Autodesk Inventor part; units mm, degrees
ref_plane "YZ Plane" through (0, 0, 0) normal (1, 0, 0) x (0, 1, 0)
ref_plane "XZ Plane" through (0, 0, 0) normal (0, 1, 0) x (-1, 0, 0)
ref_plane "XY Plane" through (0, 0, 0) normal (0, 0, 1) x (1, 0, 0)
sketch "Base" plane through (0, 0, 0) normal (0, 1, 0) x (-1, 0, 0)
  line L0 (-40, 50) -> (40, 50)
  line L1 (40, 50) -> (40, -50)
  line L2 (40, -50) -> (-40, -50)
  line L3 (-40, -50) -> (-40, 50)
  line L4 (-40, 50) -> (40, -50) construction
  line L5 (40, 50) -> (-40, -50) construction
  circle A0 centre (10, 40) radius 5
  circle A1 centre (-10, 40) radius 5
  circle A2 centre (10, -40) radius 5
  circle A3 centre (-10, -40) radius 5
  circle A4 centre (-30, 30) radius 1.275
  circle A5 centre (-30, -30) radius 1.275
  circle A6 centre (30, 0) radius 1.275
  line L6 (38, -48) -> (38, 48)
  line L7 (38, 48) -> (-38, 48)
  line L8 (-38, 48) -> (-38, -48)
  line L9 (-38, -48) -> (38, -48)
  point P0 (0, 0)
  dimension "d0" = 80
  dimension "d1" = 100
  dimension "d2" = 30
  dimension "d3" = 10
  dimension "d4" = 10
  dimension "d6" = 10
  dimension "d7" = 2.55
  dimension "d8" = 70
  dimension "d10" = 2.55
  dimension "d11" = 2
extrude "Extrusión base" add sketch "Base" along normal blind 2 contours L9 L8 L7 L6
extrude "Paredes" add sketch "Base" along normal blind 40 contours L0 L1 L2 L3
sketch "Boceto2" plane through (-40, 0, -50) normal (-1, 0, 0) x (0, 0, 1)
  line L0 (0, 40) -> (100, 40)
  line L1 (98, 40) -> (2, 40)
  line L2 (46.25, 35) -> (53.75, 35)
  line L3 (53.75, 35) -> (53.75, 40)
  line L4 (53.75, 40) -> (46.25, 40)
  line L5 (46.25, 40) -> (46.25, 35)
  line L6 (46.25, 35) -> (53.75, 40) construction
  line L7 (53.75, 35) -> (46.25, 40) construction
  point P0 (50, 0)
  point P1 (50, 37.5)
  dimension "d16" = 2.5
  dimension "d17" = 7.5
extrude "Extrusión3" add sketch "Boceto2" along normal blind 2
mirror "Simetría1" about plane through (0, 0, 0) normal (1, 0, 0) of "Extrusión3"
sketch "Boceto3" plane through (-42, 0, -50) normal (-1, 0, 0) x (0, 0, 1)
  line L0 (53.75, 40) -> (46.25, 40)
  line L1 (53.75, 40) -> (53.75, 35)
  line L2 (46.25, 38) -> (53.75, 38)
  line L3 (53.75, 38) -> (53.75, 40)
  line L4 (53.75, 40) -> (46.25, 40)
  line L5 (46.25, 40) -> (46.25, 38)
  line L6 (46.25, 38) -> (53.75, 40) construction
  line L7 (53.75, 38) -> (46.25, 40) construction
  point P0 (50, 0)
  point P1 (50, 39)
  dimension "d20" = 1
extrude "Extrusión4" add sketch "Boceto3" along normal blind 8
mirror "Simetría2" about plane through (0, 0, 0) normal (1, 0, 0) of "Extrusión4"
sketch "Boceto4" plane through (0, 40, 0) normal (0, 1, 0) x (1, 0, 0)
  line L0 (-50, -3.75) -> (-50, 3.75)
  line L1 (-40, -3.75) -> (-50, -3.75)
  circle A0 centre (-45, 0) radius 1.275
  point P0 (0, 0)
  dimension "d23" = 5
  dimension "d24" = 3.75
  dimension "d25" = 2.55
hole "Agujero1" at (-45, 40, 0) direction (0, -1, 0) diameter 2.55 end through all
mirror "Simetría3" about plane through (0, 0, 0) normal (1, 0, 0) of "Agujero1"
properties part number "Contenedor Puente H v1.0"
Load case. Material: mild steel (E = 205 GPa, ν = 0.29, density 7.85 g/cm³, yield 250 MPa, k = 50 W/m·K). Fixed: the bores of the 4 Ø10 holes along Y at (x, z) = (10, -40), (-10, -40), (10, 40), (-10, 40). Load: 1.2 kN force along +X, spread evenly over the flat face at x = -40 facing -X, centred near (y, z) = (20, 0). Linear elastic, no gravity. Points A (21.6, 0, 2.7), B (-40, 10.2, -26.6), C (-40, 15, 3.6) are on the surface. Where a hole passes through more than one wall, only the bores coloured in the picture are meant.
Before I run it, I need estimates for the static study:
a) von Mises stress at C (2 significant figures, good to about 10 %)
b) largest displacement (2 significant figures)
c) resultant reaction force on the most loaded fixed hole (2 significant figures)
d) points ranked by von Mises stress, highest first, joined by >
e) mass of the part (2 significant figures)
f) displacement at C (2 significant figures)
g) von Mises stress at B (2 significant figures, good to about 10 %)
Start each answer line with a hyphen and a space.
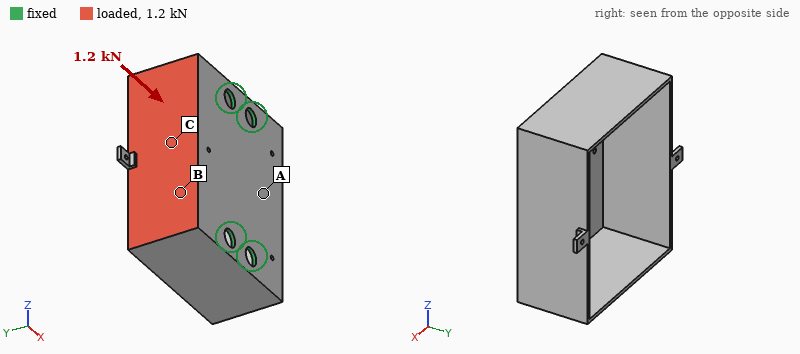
- 36 MPa
- 0.43 mm
- 560 N
- B > C > A
- 330 g
- 0.14 mm
- 79 MPa
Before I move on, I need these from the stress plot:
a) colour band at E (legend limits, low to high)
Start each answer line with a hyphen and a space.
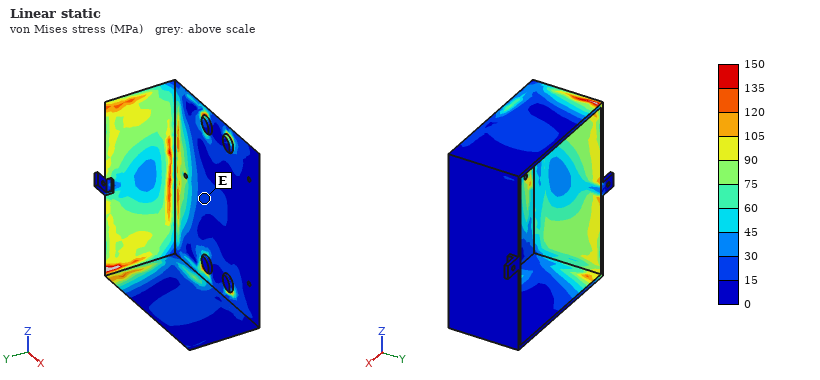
- 15 to 30 MPa
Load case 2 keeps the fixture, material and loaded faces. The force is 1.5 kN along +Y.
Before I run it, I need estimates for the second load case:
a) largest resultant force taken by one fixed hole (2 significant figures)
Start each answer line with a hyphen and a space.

- 1.5 kN
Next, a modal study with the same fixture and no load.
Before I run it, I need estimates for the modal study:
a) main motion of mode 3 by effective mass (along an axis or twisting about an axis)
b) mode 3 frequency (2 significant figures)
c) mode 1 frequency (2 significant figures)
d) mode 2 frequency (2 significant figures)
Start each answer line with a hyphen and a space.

- along Z
- 1900 Hz
- 1300 Hz
- 1300 Hz
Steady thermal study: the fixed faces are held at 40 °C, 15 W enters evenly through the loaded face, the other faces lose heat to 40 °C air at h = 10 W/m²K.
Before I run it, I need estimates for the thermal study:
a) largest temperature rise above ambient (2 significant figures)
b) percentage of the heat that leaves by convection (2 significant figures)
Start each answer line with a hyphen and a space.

- 44 K
- 28 %
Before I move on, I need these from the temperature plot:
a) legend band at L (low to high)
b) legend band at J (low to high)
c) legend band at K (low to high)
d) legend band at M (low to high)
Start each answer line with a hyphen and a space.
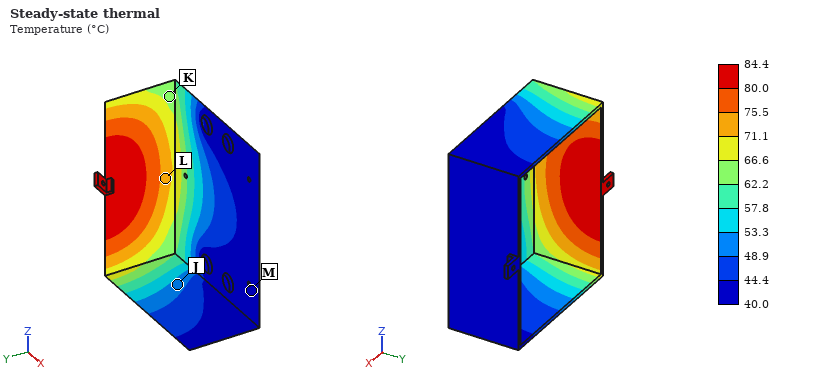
- 71.1 to 75.5 °C
- 48.9 to 53.3 °C
- 62.2 to 66.6 °C
- 40.0 to 44.4 °C
